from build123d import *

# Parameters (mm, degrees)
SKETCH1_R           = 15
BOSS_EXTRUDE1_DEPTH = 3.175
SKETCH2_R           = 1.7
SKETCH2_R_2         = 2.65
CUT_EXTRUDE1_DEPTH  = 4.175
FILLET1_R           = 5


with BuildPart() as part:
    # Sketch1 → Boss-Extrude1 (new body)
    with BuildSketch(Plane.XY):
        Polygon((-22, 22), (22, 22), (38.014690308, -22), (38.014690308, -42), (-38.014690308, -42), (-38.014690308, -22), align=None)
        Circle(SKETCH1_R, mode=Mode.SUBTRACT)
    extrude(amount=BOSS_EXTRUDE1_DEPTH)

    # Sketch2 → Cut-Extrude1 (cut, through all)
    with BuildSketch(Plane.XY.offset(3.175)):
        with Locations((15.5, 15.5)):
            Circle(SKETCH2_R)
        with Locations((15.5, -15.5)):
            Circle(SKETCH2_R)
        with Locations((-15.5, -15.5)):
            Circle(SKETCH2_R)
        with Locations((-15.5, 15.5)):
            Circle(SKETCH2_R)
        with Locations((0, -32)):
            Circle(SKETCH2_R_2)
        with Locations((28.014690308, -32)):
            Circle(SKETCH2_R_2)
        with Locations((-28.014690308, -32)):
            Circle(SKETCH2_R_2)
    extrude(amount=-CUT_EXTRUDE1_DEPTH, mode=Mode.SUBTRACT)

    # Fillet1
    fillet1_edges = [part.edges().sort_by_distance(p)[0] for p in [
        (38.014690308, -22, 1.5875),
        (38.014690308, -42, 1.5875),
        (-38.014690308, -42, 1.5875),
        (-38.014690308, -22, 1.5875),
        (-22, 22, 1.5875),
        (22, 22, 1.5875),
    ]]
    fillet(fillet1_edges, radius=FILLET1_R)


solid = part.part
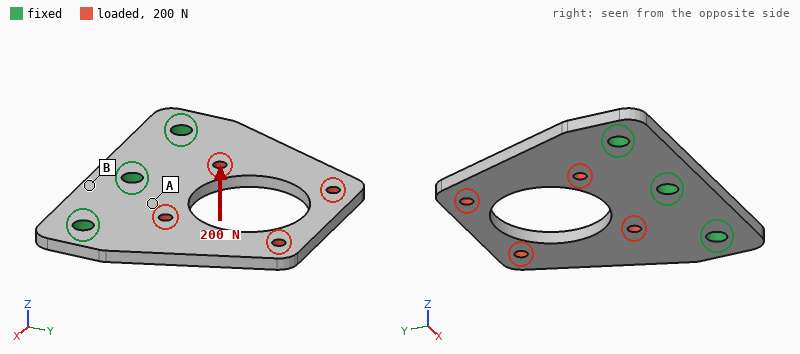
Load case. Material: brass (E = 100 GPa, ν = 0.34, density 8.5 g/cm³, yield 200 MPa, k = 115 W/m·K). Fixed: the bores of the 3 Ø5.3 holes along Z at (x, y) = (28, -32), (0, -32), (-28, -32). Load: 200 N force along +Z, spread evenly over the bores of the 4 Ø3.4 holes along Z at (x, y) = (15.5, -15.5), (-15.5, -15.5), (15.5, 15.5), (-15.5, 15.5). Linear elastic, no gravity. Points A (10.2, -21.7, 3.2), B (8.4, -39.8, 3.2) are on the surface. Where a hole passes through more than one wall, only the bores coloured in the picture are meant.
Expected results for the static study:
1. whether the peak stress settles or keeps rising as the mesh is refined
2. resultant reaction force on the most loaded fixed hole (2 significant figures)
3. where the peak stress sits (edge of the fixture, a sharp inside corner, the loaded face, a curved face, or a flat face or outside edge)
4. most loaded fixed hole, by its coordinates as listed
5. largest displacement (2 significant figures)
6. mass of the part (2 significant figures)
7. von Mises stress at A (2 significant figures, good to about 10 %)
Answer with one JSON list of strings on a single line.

["keeps rising", "95 N", "edge of the fixture", "(0, -32)", "0.33 mm", "90 g", "30 MPa"]
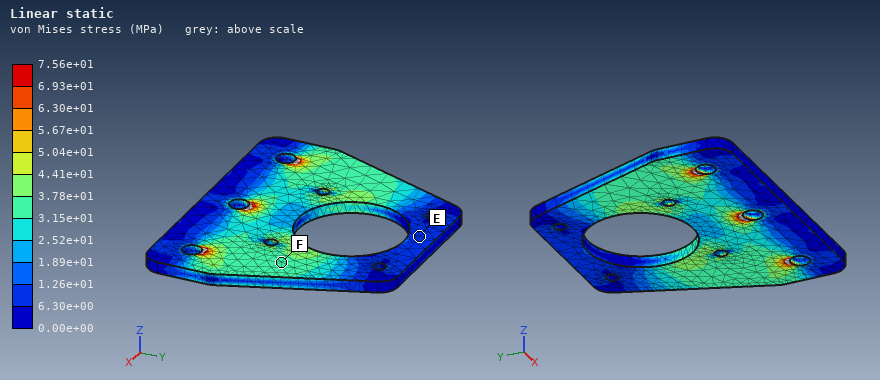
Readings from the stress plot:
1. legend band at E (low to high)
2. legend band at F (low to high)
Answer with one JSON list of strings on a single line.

["6.30e+00 to 1.26e+01 MPa", "3.15e+01 to 3.78e+01 MPa"]
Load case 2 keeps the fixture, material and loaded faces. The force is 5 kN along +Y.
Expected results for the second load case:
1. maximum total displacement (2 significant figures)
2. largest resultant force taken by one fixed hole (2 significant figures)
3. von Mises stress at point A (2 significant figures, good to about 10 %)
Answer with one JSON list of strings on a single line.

["19 µm", "1.9 kN", "23 MPa"]
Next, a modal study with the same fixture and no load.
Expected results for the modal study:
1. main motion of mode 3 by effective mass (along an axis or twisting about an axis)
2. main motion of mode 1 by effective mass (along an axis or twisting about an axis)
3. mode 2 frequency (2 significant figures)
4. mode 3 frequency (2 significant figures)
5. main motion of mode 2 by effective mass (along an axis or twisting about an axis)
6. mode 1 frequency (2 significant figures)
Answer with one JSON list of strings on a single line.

["along Z", "along Z", "1600 Hz", "3400 Hz", "twisting about Y", "760 Hz"]
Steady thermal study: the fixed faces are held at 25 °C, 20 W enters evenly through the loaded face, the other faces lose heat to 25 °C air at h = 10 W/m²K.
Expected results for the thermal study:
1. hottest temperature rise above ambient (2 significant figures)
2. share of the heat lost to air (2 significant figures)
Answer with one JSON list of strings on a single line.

["43 K", "5.8 %"]
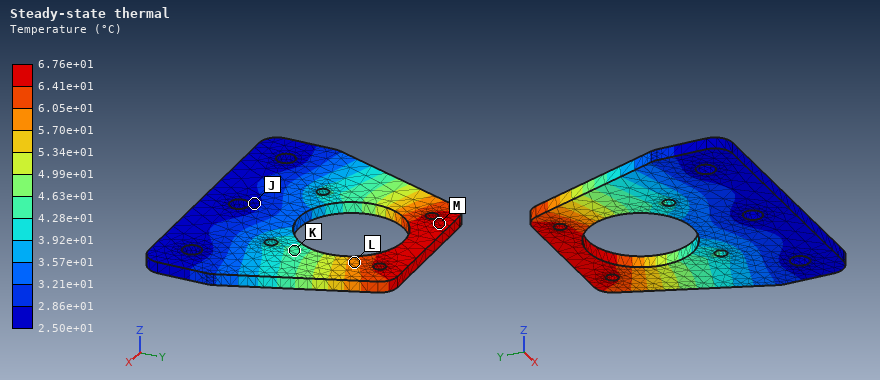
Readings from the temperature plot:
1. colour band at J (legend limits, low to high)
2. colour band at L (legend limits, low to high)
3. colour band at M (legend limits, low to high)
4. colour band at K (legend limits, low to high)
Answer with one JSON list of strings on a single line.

["2.50e+01 to 2.86e+01 °C", "5.70e+01 to 6.05e+01 °C", "6.41e+01 to 6.76e+01 °C", "4.28e+01 to 4.63e+01 °C"]
